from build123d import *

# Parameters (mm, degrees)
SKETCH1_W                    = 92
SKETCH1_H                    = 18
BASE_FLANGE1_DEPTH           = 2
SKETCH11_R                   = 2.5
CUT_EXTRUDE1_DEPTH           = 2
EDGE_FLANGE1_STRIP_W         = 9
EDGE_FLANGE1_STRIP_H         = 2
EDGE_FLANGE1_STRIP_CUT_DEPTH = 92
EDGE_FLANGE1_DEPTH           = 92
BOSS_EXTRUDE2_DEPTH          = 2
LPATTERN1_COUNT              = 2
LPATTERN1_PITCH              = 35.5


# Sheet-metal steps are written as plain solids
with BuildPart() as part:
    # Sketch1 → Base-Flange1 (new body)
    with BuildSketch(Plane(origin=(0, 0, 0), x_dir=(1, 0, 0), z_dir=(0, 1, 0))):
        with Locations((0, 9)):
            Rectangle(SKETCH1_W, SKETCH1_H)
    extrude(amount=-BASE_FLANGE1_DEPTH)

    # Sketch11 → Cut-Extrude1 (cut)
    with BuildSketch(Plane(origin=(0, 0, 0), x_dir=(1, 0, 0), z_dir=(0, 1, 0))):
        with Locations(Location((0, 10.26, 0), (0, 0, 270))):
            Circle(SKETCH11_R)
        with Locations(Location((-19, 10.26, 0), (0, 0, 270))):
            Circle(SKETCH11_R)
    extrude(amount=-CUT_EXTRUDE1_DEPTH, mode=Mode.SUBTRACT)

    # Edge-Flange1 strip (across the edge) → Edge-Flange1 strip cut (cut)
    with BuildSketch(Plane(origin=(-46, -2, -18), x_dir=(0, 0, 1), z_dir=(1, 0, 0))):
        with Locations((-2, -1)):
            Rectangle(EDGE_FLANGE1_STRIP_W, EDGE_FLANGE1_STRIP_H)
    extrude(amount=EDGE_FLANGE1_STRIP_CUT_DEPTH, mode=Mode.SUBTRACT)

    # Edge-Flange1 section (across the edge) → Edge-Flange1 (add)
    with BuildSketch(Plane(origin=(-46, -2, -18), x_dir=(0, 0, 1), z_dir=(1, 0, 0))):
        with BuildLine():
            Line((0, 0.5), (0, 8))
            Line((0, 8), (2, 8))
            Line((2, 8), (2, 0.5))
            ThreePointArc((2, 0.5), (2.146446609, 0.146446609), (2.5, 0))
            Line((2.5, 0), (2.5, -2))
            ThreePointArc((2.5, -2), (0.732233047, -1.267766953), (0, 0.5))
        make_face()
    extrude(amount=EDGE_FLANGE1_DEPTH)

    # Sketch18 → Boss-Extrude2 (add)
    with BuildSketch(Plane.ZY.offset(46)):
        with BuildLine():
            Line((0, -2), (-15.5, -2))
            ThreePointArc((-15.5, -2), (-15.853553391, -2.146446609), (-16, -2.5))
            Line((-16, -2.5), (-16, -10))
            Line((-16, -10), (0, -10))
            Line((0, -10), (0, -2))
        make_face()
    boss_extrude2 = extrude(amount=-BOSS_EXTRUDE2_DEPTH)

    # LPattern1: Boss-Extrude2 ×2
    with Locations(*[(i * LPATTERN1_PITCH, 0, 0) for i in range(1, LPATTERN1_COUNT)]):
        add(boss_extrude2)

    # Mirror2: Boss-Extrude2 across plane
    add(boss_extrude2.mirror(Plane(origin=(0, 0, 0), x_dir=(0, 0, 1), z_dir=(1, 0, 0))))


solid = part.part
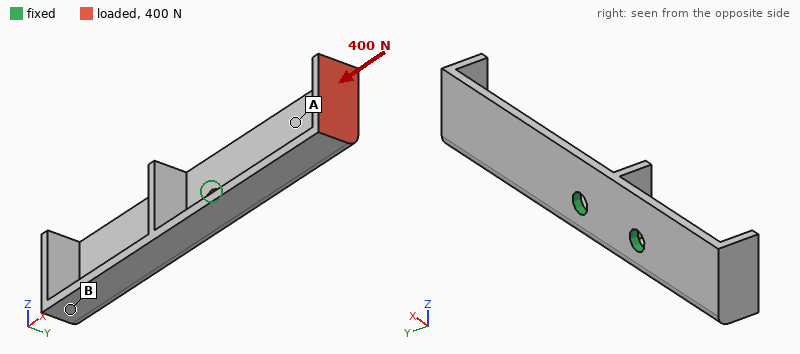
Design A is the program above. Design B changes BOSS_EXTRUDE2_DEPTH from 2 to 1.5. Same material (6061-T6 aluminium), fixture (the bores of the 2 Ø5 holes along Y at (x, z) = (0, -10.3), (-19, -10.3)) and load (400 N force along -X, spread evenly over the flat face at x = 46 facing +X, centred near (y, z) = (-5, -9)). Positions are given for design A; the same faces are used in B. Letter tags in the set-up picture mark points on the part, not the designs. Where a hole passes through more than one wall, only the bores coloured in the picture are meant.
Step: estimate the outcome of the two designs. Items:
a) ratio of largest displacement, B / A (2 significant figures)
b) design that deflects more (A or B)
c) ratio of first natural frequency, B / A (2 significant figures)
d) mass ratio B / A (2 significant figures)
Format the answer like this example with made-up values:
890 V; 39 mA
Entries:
1.2; B; 1.0; 0.96
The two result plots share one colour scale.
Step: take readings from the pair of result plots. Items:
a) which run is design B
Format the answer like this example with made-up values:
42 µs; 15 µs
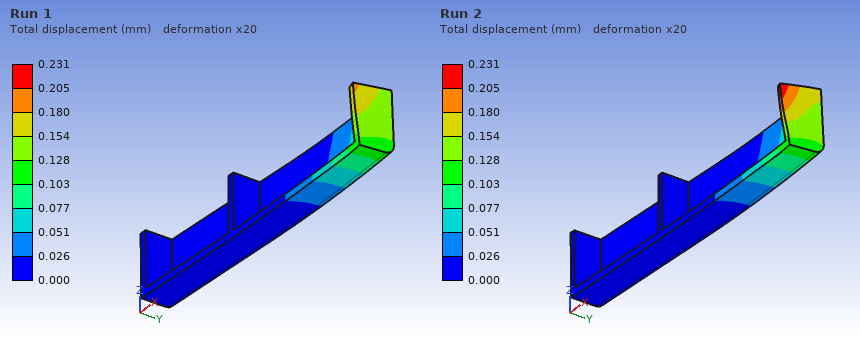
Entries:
Run 2
